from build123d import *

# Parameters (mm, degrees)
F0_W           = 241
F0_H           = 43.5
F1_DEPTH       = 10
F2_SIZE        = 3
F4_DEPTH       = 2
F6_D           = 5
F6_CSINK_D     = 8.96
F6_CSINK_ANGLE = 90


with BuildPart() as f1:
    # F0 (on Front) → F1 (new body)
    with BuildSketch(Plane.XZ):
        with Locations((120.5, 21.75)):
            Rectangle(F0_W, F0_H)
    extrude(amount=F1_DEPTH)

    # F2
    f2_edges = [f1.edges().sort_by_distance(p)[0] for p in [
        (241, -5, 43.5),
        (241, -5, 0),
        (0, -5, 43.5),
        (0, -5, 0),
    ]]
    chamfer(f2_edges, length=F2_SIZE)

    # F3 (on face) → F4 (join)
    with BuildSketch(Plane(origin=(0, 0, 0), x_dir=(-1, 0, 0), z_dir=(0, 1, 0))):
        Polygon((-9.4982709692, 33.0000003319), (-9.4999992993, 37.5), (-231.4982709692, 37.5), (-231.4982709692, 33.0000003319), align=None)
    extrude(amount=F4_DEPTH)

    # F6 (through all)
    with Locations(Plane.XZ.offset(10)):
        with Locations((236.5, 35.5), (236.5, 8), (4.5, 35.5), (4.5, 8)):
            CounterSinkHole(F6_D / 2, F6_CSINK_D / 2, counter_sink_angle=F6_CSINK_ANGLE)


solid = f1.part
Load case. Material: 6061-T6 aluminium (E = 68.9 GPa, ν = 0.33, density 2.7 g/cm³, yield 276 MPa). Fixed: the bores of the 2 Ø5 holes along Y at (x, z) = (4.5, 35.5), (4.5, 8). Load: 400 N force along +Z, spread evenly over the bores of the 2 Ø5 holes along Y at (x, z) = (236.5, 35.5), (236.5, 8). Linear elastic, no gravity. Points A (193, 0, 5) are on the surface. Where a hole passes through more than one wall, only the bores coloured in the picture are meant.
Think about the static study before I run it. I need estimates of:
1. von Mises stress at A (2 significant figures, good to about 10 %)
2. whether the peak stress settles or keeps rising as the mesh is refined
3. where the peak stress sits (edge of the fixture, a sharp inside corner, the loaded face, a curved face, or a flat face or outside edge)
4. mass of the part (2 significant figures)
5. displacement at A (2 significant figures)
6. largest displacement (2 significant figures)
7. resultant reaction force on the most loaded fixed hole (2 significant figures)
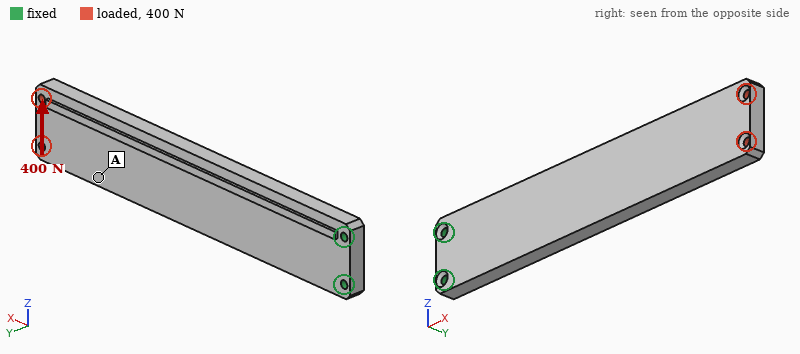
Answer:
4.7 MPa
keeps rising
edge of the fixture
290 g
0.28 mm
0.39 mm
3.1 kN
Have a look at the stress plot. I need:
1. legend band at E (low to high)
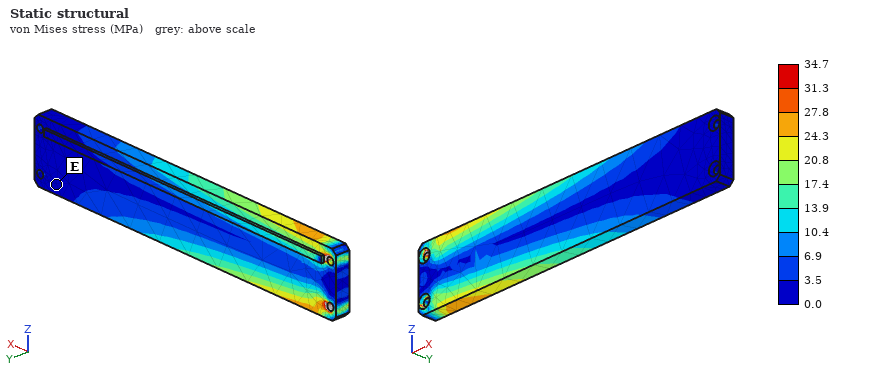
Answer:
0.0 to 3.5 MPa
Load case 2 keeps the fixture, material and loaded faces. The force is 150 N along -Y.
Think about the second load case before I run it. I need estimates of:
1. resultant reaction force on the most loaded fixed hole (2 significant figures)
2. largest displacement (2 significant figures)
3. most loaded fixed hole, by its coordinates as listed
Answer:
83 N
2.5 mm
(4.5, 8)
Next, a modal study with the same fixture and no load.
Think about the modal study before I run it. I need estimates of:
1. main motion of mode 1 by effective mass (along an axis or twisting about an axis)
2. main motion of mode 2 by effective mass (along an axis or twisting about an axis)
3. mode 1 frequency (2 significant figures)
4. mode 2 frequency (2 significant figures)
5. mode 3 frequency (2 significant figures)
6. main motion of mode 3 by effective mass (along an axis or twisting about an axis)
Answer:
along Y
along Z
150 Hz
610 Hz
910 Hz
along Y
